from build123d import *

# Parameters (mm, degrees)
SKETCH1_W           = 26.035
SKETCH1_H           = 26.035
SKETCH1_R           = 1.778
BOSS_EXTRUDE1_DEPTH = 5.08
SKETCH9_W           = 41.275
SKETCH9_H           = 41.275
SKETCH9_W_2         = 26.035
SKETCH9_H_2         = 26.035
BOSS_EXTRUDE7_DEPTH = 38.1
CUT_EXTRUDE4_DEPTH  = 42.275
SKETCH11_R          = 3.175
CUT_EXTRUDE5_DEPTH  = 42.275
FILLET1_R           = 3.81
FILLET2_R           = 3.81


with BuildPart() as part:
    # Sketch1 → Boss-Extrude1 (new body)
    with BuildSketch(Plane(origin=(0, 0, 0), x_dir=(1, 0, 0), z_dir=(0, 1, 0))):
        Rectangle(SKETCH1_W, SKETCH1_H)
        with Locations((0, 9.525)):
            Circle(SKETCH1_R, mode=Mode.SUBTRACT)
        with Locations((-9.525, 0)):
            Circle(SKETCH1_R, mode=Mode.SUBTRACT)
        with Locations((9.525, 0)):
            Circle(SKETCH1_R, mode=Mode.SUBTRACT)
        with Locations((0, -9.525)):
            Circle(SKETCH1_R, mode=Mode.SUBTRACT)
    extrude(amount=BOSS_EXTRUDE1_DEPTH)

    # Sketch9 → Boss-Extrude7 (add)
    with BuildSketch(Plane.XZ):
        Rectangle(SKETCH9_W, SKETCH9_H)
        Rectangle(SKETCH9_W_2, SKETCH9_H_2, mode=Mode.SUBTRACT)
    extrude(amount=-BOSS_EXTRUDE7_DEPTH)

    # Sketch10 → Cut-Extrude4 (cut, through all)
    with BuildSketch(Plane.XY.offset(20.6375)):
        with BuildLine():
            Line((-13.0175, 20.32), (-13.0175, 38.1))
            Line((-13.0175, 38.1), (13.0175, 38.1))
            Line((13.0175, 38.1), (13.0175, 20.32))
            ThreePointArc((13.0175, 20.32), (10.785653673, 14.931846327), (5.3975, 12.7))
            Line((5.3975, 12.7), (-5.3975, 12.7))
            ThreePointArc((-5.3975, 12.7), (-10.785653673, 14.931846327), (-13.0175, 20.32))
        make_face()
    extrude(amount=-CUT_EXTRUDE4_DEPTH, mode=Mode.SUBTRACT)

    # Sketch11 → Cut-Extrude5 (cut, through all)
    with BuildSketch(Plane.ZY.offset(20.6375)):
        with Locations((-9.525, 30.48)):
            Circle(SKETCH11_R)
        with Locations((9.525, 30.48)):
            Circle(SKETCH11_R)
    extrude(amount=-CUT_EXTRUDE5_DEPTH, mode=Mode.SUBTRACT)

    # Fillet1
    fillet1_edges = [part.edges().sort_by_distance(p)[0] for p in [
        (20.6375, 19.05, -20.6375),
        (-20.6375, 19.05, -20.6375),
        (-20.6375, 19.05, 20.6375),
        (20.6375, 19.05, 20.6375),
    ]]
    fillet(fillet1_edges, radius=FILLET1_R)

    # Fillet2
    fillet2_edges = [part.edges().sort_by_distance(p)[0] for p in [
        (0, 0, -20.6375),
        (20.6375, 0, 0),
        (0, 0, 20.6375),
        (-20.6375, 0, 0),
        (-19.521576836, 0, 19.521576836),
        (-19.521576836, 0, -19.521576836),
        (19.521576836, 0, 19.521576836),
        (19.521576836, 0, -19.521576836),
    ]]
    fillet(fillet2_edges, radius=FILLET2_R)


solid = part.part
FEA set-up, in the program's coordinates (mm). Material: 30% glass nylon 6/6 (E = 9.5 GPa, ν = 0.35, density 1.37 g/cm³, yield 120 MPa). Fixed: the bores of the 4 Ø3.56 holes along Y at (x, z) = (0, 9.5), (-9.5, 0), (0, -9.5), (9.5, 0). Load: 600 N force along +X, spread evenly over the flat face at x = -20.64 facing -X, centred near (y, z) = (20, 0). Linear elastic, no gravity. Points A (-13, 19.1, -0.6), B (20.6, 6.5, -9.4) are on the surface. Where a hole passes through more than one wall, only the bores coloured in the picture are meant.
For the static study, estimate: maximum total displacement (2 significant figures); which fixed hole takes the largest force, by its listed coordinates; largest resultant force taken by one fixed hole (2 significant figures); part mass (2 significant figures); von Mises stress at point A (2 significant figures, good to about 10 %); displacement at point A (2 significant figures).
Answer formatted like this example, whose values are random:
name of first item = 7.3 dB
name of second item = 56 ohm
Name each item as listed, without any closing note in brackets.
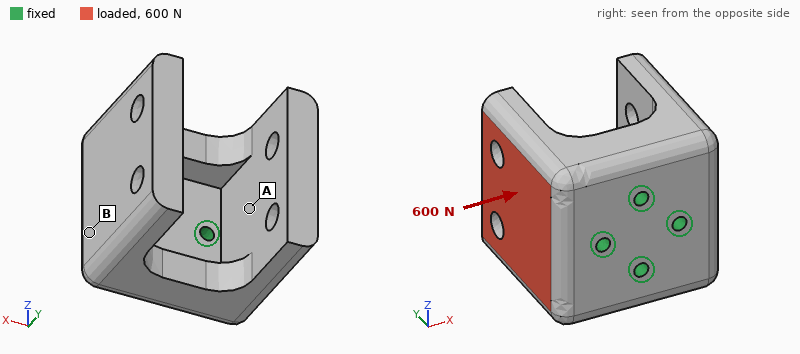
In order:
maximum total displacement = 0.27 mm
which fixed hole takes the largest force, by its listed coordinates = (-9.5, 0)
largest resultant force taken by one fixed hole = 470 N
part mass = 42 g
von Mises stress at point A = 5.9 MPa
displacement at point A = 0.10 mm
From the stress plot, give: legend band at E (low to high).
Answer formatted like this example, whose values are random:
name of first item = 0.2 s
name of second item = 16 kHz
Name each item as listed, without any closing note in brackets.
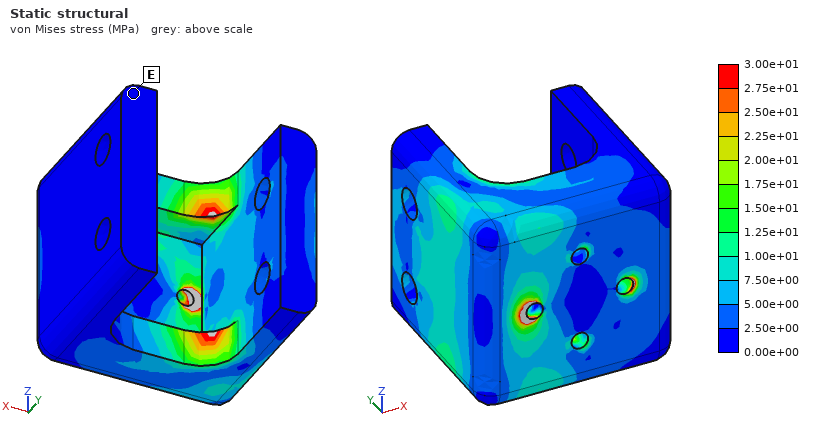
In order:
legend band at E = 0.00e+00 to 2.50e+00 MPa
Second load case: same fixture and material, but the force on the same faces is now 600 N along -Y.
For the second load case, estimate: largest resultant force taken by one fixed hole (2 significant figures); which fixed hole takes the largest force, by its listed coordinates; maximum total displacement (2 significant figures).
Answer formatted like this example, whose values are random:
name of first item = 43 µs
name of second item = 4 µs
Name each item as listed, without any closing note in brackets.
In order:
largest resultant force taken by one fixed hole = 690 N
which fixed hole takes the largest force, by its listed coordinates = (-9.5, 0)
maximum total displacement = 0.16 mm
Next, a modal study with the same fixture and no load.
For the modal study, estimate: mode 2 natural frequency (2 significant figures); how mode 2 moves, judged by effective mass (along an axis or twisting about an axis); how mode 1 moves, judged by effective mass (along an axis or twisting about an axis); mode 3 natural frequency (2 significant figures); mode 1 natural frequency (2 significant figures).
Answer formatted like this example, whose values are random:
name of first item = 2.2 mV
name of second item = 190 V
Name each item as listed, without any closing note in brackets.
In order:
mode 2 natural frequency = 2600 Hz
how mode 2 moves, judged by effective mass = along Z
how mode 1 moves, judged by effective mass = along X
mode 3 natural frequency = 2800 Hz
mode 1 natural frequency = 2300 Hz
